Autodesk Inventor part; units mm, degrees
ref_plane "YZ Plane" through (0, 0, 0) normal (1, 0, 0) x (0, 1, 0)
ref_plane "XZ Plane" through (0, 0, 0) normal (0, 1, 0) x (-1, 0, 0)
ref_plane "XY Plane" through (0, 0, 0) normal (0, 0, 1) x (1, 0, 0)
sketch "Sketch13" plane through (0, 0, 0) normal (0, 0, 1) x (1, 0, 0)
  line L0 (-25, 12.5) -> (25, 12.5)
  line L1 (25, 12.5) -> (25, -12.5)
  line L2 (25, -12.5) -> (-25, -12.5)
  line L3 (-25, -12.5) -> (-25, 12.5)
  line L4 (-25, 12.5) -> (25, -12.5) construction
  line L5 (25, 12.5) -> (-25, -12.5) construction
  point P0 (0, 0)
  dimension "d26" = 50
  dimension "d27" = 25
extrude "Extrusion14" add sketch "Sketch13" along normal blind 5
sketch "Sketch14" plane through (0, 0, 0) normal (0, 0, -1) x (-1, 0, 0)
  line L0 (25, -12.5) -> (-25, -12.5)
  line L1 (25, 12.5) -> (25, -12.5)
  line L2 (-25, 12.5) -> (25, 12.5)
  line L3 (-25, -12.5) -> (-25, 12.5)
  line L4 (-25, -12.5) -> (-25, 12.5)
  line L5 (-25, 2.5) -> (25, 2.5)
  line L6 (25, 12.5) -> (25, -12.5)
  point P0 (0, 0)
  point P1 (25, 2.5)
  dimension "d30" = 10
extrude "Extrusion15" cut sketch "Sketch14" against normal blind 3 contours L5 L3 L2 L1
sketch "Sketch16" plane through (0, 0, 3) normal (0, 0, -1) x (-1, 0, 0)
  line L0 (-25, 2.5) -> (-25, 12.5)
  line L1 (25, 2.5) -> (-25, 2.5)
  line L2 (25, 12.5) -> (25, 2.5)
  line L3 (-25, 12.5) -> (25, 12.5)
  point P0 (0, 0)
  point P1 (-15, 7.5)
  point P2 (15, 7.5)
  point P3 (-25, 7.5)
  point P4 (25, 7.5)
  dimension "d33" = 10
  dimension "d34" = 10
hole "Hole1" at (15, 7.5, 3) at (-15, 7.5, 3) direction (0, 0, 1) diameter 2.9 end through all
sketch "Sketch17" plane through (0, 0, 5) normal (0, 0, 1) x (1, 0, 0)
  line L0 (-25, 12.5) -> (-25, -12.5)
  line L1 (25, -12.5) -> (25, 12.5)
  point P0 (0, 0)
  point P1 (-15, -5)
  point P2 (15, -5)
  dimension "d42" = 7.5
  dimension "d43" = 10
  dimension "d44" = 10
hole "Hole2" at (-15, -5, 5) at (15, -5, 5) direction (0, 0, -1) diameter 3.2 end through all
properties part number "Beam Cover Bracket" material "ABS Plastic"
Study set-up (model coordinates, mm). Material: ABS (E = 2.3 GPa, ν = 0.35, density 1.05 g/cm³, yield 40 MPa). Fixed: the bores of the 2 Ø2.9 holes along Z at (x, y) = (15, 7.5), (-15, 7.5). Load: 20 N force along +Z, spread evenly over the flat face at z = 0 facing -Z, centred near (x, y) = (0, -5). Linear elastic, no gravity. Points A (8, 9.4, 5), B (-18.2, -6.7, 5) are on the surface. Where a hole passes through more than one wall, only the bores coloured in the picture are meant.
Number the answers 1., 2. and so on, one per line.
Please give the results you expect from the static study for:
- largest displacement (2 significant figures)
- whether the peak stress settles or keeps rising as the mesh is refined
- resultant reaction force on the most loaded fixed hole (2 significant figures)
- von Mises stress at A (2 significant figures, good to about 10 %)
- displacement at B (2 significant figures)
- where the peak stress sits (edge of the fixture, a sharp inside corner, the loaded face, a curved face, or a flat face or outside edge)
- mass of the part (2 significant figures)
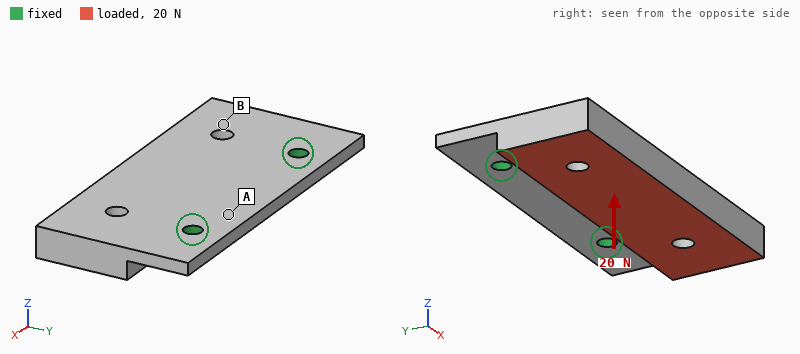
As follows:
1. 0.35 mm
2. keeps rising
3. 10 N
4. 2.6 MPa
5. 0.22 mm
6. edge of the fixture
7. 4.9 g
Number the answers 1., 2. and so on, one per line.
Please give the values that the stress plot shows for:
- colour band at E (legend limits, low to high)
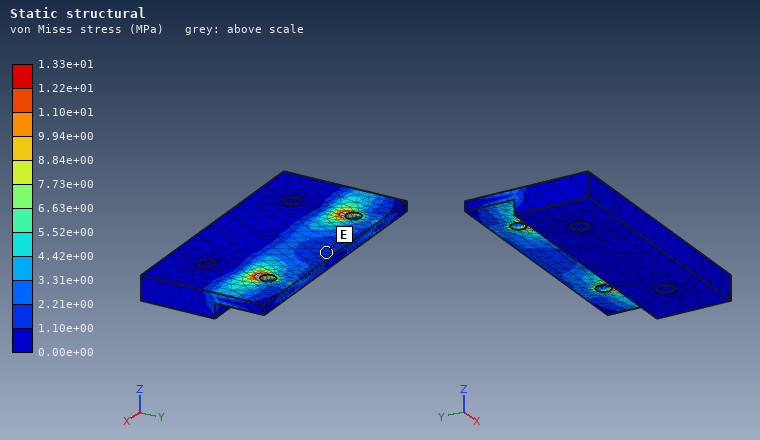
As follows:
1. 1.10e+00 to 2.21e+00 MPa
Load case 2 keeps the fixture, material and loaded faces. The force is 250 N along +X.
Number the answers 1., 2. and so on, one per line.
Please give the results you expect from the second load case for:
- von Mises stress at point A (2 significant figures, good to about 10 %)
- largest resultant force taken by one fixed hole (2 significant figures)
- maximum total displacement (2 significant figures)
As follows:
1. 2.6 MPa
2. 160 N
3. 0.21 mm
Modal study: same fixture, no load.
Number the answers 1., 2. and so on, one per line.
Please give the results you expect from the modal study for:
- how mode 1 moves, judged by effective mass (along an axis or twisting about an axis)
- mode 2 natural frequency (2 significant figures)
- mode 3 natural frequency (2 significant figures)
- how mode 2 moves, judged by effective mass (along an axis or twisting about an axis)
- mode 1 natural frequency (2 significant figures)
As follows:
1. along Z
2. 1900 Hz
3. 3400 Hz
4. twisting about Y
5. 740 Hz
